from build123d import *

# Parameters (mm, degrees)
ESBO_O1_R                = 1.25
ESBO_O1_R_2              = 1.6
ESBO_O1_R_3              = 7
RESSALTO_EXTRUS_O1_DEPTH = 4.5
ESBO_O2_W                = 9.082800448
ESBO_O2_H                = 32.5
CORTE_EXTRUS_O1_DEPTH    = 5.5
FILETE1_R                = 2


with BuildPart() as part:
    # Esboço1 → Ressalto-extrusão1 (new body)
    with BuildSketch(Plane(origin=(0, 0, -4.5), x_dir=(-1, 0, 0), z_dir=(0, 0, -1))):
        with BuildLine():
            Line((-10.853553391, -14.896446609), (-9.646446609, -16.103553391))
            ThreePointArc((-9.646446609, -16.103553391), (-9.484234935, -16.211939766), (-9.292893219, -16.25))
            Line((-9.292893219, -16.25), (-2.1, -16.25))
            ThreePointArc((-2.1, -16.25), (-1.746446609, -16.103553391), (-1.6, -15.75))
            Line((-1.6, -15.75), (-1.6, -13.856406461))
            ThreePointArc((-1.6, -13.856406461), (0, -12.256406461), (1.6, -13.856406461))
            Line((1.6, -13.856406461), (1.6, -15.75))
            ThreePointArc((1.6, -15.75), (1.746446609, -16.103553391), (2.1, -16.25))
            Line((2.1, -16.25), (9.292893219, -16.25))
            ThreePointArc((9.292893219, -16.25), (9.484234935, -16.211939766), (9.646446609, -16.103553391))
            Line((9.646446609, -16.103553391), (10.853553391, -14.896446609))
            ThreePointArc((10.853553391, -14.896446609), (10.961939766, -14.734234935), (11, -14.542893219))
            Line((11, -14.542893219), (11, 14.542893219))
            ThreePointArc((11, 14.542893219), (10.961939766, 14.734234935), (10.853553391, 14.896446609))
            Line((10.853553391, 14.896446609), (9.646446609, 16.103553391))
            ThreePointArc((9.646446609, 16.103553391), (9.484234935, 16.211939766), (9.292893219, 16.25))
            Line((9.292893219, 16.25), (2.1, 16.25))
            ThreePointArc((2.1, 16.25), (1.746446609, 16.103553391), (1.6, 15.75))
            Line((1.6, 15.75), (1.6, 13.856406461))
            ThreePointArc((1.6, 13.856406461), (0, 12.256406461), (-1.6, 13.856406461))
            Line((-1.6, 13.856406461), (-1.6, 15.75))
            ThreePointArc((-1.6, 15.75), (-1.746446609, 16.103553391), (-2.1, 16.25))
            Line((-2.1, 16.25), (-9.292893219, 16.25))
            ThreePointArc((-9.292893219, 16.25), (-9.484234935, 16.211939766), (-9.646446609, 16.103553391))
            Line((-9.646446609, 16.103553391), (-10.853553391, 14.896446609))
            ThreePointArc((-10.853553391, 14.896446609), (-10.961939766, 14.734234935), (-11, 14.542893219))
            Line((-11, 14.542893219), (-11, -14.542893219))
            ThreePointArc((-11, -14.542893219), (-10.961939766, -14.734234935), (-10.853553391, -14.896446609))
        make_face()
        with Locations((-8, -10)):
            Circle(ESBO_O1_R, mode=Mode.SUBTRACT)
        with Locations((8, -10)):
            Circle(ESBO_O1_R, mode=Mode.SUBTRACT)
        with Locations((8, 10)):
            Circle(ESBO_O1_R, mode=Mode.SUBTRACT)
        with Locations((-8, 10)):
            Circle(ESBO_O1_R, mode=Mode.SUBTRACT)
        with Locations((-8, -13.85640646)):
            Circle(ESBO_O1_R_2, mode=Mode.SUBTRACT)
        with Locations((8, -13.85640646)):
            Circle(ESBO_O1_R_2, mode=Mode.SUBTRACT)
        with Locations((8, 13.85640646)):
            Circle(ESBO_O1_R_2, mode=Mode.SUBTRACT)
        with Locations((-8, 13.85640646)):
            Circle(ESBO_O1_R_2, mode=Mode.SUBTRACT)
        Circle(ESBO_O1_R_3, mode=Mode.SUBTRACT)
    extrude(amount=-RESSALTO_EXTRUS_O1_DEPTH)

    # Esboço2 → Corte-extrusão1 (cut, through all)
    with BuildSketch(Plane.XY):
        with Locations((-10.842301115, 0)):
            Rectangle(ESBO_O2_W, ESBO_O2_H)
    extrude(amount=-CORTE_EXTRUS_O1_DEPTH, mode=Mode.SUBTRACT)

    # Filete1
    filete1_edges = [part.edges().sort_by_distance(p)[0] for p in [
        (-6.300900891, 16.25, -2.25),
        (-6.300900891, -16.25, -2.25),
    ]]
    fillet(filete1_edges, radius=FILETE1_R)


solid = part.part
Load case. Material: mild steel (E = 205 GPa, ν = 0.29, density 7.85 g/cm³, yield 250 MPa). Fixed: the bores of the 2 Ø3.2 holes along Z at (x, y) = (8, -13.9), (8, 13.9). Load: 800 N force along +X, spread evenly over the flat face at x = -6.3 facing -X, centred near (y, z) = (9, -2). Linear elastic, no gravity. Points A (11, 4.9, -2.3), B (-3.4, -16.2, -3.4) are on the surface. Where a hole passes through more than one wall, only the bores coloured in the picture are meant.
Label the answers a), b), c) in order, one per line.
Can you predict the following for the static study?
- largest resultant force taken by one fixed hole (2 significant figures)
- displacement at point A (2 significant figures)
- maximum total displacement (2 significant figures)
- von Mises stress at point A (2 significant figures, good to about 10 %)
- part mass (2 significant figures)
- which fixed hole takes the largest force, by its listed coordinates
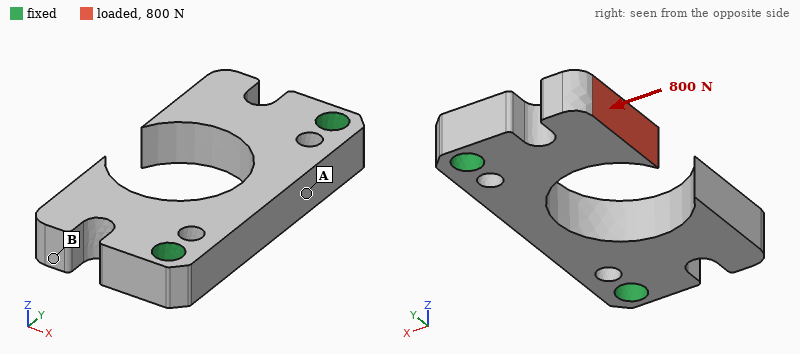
a) 700 N
b) 3.7 µm
c) 22 µm
d) 38 MPa
e) 13 g
f) (8, 13.9)
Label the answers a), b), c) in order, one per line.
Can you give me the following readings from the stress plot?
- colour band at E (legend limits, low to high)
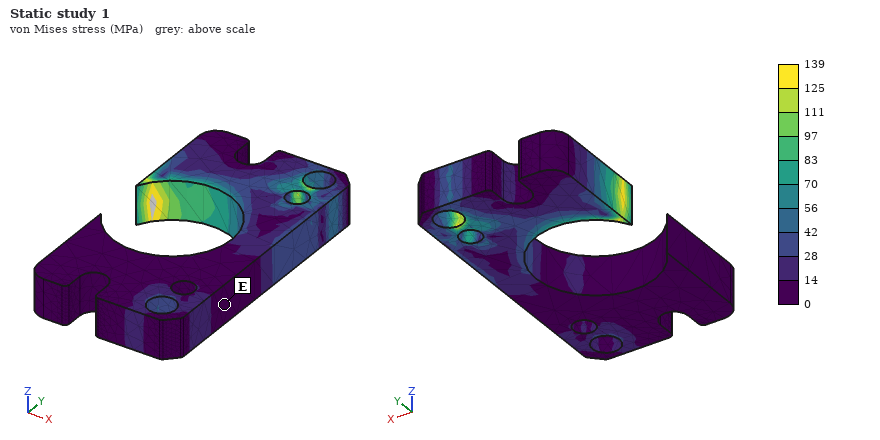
a) 0 to 14 MPa
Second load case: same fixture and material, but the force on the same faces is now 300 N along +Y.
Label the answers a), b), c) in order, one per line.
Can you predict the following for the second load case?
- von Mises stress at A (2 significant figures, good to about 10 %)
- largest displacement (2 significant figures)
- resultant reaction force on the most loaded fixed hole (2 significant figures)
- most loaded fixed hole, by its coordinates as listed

a) 36 MPa
b) 20 µm
c) 340 N
d) (8, 13.9)
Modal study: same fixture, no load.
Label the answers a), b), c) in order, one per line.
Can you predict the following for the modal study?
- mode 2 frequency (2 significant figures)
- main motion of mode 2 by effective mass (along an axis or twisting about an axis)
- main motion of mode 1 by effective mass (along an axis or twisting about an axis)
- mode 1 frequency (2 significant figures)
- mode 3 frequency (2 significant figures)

a) 15 kHz
b) twisting about X
c) along Z
d) 14 kHz
e) 16 kHz
